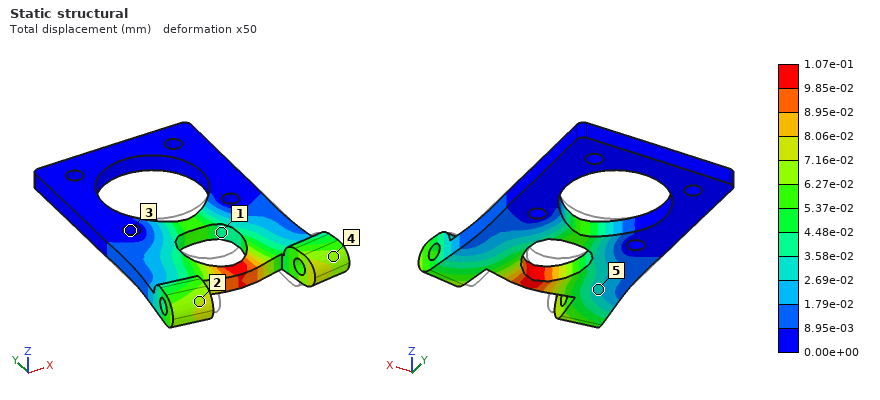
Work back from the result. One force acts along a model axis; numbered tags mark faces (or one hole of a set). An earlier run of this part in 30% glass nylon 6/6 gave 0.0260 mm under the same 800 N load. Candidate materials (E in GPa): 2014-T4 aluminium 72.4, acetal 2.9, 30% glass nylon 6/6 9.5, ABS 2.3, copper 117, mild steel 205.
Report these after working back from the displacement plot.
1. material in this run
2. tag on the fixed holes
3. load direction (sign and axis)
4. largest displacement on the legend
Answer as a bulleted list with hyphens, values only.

- ABS
- 3
- -Y
- 1.07e-01 mm
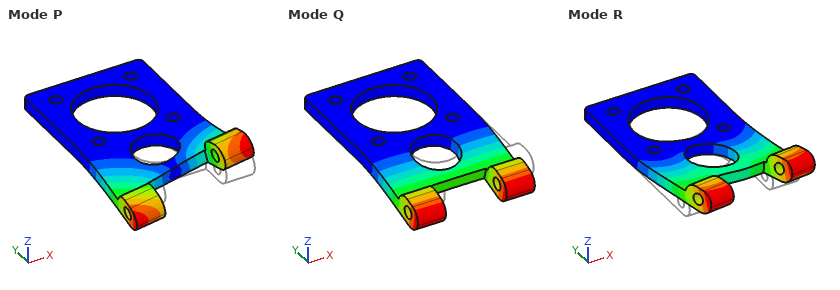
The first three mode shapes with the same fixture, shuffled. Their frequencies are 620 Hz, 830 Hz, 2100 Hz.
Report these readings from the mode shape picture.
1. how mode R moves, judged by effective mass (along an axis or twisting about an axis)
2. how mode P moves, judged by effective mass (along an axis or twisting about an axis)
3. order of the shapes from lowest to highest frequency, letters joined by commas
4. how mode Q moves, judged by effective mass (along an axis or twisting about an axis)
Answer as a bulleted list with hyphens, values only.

- along X
- twisting about Y
- Q, P, R
- along Z
